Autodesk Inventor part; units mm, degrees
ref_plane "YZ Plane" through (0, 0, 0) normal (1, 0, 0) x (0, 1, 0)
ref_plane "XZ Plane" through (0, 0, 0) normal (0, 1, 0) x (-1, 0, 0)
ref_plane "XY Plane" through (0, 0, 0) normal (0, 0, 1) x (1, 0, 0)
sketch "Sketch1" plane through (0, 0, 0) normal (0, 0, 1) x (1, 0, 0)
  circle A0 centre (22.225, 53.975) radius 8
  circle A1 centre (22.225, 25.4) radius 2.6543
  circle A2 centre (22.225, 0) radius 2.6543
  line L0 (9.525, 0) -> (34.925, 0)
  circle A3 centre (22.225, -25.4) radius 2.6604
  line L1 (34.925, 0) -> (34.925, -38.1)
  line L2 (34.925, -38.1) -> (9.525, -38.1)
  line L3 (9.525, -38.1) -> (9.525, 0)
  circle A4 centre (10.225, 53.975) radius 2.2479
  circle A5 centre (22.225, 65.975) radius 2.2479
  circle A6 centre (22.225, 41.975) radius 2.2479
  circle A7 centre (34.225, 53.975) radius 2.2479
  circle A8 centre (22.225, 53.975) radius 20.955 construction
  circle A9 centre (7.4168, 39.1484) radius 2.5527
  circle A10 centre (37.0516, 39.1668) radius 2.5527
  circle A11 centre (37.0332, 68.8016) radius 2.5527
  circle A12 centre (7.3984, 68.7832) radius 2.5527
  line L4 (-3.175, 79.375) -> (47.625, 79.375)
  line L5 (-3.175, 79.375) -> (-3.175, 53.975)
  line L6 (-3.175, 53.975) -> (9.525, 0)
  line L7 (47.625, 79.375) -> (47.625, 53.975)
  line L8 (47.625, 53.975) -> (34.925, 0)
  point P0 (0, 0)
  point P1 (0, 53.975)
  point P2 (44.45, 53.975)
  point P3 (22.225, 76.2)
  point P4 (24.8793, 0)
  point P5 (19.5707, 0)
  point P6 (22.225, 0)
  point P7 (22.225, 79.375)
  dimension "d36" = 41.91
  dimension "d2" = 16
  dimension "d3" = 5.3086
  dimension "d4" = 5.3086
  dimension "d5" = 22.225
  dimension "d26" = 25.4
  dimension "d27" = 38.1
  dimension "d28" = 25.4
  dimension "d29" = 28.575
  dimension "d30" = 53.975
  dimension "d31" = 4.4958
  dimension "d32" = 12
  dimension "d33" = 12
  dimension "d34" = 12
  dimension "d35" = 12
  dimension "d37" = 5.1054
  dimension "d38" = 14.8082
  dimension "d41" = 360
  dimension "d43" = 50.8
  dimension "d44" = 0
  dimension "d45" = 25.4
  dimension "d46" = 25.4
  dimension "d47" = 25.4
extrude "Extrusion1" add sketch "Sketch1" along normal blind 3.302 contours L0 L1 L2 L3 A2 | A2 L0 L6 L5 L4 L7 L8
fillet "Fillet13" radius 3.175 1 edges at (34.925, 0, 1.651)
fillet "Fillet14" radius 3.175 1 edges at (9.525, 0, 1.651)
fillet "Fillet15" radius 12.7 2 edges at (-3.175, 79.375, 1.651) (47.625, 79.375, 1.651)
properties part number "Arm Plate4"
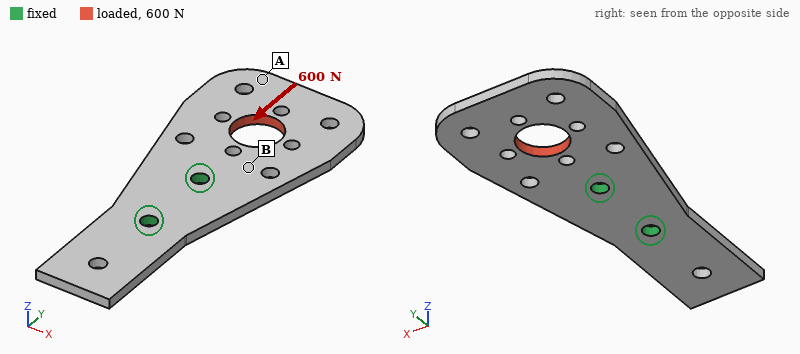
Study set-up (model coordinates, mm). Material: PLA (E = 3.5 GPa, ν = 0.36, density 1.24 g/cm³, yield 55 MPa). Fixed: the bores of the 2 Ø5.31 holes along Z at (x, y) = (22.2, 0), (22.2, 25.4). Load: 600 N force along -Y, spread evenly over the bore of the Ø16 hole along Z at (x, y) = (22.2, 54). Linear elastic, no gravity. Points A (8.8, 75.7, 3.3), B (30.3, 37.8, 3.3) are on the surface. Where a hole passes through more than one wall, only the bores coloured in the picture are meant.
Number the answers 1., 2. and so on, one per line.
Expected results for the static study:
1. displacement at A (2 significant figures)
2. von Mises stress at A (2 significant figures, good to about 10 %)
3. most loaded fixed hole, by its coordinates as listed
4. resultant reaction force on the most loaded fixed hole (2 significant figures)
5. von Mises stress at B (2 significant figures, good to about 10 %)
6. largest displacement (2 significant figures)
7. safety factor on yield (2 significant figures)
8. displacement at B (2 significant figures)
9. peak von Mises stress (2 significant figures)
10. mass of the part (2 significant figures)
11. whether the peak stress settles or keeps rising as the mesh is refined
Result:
1. 0.076 mm
2. 1.9 MPa
3. (22.2, 25.4)
4. 450 N
5. 6.3 MPa
6. 0.11 mm
7. 2.7
8. 0.033 mm
9. 20 MPa
10. 16 g
11. settles
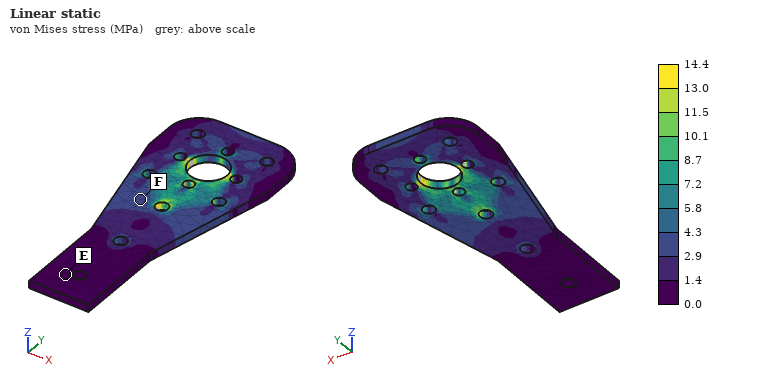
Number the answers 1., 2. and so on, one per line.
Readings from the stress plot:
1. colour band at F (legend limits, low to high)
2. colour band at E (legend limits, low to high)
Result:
1. 2.9 to 4.3 MPa
2. 0.0 to 1.4 MPa
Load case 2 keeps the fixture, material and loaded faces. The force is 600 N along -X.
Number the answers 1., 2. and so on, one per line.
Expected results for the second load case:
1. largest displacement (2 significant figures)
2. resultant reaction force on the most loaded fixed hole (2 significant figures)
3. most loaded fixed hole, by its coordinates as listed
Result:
1. 0.93 mm
2. 1.1 kN
3. (22.2, 25.4)
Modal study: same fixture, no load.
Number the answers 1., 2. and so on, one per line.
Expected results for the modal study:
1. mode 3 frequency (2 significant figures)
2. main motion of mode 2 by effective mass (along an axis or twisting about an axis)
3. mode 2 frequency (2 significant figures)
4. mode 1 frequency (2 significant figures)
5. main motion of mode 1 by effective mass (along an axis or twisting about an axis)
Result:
1. 660 Hz
2. twisting about Y
3. 570 Hz
4. 280 Hz
5. along Z
